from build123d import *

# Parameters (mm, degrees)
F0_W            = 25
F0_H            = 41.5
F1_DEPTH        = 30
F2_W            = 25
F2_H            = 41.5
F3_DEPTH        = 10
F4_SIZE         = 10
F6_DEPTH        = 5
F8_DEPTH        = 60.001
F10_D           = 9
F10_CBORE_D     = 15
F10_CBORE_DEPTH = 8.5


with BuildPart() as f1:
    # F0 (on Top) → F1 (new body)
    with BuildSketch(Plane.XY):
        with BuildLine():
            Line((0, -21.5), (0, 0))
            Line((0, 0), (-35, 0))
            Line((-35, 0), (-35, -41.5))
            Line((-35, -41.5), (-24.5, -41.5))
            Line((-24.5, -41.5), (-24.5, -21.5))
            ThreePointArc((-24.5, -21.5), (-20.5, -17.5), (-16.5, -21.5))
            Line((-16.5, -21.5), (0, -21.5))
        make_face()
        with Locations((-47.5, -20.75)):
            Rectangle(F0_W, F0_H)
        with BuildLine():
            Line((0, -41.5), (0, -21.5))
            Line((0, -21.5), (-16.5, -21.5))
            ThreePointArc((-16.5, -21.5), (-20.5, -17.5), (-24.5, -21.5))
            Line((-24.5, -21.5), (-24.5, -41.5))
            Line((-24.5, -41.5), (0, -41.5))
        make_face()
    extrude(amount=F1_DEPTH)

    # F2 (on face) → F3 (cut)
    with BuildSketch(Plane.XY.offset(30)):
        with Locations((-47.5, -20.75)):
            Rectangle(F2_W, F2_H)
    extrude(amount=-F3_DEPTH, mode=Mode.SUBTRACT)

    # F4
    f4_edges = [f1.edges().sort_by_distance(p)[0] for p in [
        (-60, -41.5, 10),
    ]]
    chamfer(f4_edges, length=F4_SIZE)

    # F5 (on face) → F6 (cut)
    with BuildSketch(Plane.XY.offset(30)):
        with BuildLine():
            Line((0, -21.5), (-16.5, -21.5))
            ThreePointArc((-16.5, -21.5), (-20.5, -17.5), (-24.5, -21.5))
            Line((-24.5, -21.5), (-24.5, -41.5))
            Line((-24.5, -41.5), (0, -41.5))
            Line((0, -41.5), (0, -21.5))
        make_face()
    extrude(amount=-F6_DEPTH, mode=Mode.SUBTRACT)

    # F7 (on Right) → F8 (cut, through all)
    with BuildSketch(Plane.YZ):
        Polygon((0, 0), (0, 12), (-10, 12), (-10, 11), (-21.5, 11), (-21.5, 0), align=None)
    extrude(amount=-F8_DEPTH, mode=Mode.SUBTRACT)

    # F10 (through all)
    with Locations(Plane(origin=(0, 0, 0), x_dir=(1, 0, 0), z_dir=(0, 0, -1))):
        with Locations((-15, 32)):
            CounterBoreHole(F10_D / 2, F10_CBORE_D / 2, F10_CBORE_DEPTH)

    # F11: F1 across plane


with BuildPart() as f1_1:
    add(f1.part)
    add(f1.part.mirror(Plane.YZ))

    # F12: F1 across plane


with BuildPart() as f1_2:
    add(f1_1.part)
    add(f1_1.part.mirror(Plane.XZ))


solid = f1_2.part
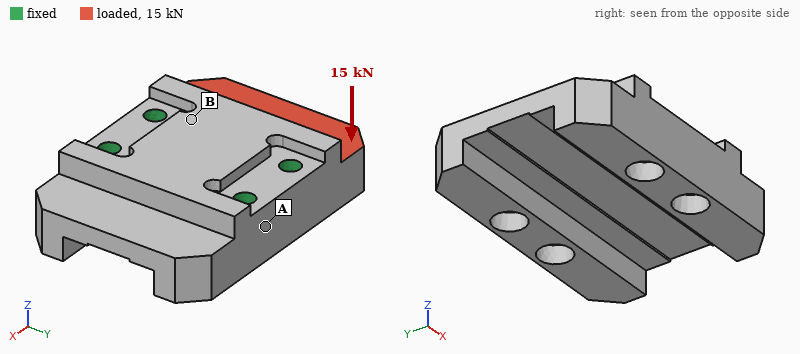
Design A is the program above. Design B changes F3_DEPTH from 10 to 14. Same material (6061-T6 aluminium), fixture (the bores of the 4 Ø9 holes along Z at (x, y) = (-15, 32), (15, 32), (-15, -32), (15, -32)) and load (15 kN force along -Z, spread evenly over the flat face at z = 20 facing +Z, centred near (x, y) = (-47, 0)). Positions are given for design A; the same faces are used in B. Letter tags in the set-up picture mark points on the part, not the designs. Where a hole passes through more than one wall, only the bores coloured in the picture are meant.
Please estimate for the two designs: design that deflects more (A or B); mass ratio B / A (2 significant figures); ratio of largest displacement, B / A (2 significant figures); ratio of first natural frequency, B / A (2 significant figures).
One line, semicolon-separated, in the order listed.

B; 0.91; 2.0; 1.1
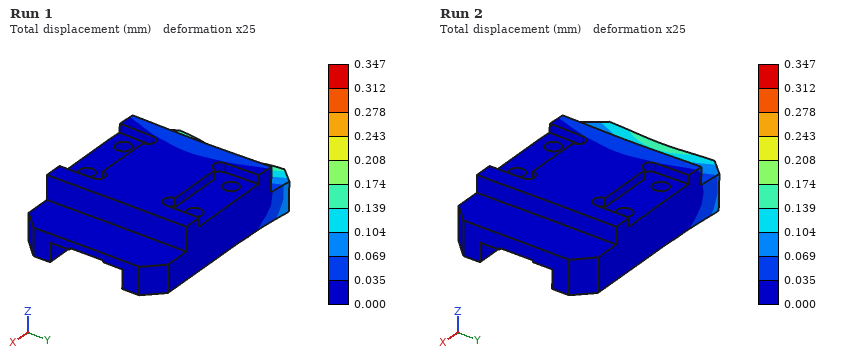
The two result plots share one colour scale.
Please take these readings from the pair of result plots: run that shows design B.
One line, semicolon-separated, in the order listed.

Run 1
